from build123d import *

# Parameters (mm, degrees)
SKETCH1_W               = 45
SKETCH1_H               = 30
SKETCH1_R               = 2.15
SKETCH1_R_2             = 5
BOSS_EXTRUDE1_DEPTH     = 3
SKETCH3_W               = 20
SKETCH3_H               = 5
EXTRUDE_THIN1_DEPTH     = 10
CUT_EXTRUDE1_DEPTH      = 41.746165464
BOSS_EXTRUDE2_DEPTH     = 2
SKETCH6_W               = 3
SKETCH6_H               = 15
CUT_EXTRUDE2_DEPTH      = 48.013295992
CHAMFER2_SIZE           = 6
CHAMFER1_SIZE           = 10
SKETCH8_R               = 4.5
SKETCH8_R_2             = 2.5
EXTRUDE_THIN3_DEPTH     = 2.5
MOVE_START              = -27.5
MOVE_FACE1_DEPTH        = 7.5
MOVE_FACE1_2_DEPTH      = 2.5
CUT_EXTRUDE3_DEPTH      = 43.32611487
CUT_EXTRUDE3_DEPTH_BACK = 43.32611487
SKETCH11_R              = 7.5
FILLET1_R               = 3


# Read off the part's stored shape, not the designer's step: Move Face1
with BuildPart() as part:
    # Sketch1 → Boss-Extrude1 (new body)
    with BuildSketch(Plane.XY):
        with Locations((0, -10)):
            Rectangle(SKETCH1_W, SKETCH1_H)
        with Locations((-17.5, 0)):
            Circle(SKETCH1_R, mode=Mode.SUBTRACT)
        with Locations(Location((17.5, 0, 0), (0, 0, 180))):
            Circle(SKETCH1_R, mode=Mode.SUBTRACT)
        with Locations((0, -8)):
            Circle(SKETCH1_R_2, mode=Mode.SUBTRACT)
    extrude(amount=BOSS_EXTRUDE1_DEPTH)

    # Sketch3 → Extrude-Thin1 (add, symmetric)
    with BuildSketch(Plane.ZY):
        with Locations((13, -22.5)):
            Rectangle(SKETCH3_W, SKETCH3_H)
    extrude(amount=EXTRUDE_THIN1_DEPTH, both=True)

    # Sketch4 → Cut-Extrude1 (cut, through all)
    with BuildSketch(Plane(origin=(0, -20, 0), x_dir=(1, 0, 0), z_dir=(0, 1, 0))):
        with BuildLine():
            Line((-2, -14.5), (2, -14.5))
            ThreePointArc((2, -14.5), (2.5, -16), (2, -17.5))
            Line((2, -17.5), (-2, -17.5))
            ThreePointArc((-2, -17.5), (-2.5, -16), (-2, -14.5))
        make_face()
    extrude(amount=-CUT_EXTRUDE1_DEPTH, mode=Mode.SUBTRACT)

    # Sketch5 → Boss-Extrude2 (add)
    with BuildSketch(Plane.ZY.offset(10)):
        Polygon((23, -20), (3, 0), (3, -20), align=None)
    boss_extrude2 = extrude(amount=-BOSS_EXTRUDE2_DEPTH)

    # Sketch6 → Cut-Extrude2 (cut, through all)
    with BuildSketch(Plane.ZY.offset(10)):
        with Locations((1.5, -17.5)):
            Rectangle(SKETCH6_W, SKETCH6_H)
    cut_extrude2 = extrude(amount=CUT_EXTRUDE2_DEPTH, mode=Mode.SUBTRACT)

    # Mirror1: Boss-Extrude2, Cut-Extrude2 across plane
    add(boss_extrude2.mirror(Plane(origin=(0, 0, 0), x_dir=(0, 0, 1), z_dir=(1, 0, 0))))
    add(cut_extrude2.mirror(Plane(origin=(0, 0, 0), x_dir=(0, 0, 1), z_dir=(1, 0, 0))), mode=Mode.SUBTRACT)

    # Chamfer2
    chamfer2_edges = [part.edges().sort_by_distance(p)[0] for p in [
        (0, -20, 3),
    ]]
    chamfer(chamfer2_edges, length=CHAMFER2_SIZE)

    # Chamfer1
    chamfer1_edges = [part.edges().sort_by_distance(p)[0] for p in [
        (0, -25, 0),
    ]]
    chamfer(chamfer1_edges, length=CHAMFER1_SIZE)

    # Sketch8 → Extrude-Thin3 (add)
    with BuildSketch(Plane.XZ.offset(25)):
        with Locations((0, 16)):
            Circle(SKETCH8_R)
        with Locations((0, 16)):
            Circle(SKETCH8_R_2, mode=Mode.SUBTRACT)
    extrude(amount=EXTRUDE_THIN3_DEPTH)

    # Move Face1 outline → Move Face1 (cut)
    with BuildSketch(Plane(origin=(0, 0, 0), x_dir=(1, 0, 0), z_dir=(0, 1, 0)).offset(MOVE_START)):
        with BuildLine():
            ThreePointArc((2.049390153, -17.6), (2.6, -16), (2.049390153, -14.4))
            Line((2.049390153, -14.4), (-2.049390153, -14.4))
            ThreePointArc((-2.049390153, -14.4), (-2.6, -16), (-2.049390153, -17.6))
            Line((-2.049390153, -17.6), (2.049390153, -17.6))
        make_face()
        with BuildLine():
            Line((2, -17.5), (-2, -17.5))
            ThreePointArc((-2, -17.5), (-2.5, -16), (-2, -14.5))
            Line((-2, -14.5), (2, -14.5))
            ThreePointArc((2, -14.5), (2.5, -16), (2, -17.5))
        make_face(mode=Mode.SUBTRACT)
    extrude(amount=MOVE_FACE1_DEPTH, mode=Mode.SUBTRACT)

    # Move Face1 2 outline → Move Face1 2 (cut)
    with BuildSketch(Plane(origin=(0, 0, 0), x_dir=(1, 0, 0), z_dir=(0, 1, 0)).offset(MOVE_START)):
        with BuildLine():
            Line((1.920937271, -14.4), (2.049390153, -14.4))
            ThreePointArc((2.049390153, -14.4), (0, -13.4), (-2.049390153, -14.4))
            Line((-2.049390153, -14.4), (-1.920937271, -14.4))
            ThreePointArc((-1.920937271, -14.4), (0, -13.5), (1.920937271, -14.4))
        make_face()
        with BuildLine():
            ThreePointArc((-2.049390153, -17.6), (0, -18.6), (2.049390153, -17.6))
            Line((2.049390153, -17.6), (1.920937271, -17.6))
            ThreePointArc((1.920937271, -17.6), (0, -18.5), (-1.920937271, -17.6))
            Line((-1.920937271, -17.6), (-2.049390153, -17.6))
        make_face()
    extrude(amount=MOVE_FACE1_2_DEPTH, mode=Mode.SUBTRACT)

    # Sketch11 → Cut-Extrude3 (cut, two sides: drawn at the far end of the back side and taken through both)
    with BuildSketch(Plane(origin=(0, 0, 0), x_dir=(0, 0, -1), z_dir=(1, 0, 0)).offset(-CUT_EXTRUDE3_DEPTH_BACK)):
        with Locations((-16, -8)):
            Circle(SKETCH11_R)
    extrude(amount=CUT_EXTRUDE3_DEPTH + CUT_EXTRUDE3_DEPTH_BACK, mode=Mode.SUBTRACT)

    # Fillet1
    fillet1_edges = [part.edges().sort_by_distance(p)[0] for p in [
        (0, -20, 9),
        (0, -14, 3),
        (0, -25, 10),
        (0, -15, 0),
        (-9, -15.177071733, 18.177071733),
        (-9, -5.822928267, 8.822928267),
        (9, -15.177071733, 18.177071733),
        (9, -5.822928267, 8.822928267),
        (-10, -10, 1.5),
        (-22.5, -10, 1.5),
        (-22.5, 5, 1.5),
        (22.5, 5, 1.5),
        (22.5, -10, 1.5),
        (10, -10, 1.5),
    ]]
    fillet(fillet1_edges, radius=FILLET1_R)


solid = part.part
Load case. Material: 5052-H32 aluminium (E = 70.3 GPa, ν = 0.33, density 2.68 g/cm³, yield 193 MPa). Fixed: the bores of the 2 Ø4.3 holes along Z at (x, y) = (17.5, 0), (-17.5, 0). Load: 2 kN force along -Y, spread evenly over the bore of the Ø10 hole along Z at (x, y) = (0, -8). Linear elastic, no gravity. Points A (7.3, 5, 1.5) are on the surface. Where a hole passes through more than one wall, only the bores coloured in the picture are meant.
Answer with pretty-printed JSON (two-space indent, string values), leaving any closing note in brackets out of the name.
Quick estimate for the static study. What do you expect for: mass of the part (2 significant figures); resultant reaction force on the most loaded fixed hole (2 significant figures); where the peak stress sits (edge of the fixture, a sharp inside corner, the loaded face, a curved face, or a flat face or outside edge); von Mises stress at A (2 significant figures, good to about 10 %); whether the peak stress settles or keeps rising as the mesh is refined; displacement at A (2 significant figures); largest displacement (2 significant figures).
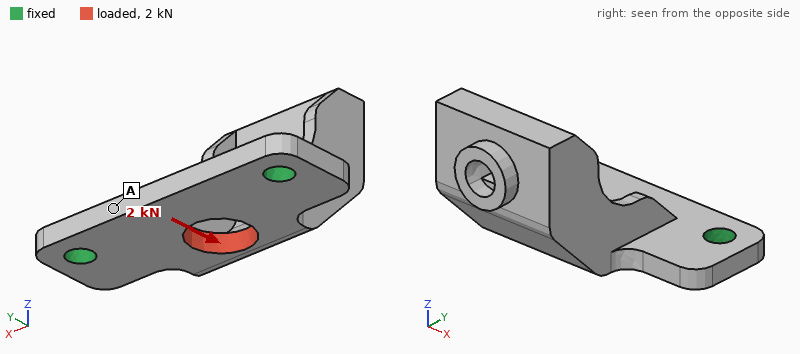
{
  "mass of the part": "12 g",
  "resultant reaction force on the most loaded fixed hole": "1.1 kN",
  "where the peak stress sits": "edge of the fixture",
  "von Mises stress at A": "26 MPa",
  "whether the peak stress settles or keeps rising as the mesh is refined": "keeps rising",
  "displacement at A": "15 µm",
  "largest displacement": "21 µm"
}
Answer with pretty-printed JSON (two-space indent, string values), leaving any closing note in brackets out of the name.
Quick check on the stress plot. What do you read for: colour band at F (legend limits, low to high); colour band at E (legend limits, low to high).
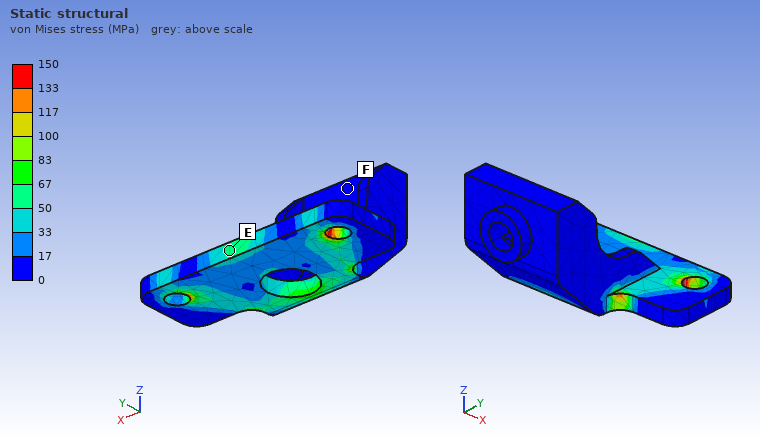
{
  "colour band at F": "0 to 17 MPa",
  "colour band at E": "50 to 67 MPa"
}
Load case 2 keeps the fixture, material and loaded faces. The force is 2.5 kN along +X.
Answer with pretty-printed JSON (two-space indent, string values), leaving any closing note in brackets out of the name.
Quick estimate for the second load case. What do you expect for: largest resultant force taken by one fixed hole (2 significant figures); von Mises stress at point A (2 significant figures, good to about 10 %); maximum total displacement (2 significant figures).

{
  "largest resultant force taken by one fixed hole": "1.3 kN",
  "von Mises stress at point A": "22 MPa",
  "maximum total displacement": "18 µm"
}
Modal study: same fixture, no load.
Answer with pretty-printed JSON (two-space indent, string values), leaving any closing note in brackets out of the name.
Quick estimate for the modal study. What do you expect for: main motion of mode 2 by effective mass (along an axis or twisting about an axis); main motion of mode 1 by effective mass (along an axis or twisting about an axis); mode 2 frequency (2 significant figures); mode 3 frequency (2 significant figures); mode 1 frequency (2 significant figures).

{
  "main motion of mode 2 by effective mass": "along X",
  "main motion of mode 1 by effective mass": "along Z",
  "mode 2 frequency": "4600 Hz",
  "mode 3 frequency": "10 kHz",
  "mode 1 frequency": "2200 Hz"
}
